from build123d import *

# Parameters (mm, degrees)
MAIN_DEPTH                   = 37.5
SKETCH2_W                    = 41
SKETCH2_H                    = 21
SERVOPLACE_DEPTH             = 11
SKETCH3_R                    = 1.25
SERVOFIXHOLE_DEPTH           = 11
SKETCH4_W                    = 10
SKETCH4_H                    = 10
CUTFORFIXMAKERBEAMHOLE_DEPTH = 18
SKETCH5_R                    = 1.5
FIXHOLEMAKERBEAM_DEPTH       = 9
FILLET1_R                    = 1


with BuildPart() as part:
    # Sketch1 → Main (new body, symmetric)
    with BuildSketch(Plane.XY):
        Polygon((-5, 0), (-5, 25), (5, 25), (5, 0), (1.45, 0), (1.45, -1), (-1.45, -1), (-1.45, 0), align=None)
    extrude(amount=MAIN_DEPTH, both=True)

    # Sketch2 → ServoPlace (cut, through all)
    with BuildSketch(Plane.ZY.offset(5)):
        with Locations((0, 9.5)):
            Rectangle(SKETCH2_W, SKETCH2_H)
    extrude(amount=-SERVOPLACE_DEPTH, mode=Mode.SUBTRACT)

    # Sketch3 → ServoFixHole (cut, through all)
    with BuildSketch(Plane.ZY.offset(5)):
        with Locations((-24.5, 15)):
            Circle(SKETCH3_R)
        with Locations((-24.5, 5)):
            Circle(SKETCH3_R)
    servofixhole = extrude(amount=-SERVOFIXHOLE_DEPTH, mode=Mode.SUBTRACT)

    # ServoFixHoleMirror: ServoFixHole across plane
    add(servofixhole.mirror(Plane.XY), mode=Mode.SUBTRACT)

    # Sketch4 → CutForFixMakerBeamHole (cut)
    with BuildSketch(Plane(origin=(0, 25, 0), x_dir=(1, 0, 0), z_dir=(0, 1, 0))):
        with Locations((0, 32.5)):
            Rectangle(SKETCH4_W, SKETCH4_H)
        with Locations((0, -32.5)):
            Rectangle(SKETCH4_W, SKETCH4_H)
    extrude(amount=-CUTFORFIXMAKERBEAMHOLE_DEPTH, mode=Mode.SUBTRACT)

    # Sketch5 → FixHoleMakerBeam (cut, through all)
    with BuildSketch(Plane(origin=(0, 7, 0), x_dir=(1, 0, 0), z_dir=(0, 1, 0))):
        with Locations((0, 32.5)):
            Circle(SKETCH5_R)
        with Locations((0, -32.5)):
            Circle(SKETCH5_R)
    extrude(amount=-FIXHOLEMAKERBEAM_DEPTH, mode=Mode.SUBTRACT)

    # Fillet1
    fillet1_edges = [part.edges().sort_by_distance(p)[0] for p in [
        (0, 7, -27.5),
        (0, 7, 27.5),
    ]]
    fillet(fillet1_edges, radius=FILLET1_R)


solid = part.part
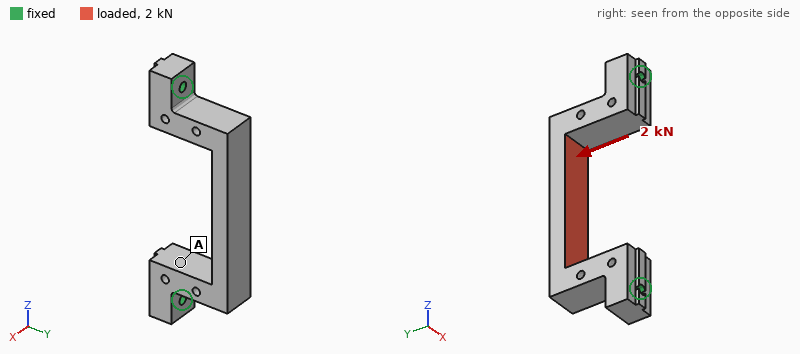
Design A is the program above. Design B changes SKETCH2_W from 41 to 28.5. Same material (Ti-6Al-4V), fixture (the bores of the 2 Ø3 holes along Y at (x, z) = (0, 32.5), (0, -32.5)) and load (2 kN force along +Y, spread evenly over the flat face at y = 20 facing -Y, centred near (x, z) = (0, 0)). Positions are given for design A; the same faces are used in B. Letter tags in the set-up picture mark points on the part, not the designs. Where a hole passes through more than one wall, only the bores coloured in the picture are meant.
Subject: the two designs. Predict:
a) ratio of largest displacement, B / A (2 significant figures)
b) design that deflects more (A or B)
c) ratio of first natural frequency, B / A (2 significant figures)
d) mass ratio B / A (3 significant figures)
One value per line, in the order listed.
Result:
0.47
A
0.95
1.38
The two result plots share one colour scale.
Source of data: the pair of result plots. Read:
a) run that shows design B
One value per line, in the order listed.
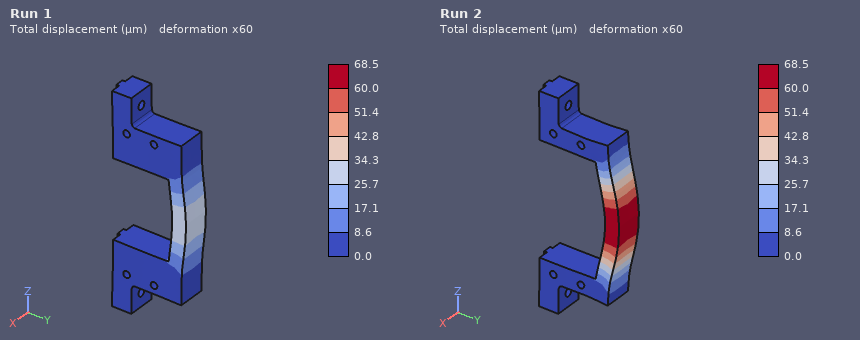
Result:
Run 1
